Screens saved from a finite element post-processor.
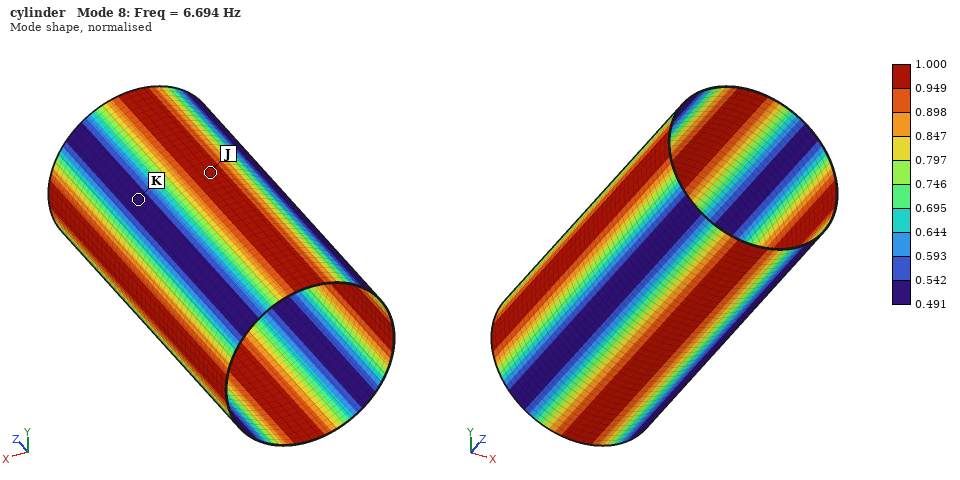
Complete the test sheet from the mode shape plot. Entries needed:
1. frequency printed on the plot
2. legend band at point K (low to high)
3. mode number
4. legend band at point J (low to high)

6.694 Hz
0.491 to 0.542
8
0.949 to 1.000
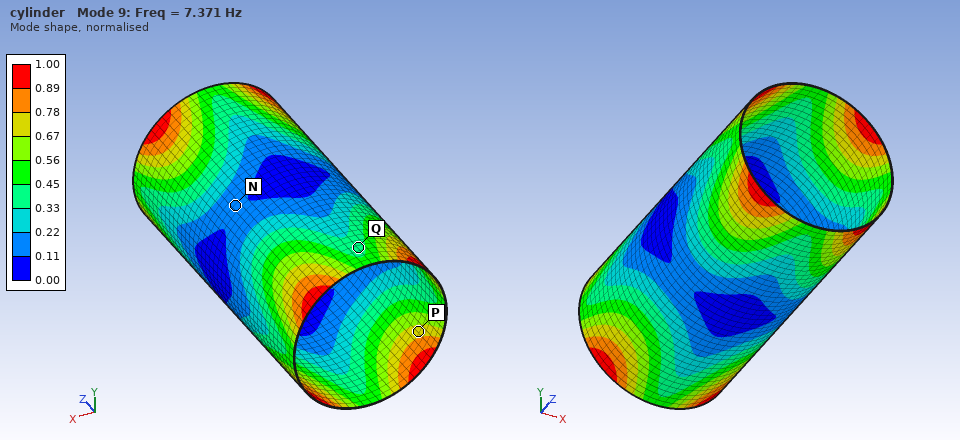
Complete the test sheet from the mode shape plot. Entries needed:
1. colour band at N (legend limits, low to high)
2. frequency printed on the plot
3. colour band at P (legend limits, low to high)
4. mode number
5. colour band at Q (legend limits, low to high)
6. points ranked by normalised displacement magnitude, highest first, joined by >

0.11 to 0.22
7.371 Hz
0.67 to 0.78
9
0.33 to 0.45
P > Q > N
